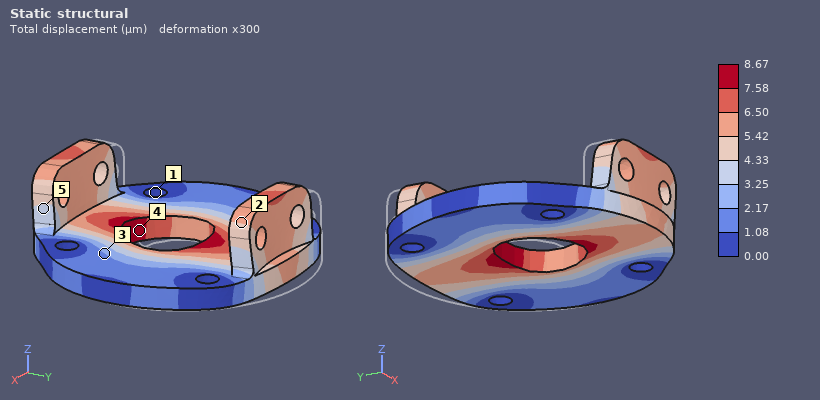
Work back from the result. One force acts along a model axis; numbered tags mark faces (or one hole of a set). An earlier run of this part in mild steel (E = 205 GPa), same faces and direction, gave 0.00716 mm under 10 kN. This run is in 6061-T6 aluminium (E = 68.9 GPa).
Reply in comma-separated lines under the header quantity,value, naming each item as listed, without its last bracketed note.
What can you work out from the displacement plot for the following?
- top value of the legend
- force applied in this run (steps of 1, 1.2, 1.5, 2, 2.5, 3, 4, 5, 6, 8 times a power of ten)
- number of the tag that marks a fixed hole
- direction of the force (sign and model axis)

quantity,value
top value of the legend,8.67 µm
force applied in this run,4 kN
number of the tag that marks a fixed hole,1
direction of the force,-Y
